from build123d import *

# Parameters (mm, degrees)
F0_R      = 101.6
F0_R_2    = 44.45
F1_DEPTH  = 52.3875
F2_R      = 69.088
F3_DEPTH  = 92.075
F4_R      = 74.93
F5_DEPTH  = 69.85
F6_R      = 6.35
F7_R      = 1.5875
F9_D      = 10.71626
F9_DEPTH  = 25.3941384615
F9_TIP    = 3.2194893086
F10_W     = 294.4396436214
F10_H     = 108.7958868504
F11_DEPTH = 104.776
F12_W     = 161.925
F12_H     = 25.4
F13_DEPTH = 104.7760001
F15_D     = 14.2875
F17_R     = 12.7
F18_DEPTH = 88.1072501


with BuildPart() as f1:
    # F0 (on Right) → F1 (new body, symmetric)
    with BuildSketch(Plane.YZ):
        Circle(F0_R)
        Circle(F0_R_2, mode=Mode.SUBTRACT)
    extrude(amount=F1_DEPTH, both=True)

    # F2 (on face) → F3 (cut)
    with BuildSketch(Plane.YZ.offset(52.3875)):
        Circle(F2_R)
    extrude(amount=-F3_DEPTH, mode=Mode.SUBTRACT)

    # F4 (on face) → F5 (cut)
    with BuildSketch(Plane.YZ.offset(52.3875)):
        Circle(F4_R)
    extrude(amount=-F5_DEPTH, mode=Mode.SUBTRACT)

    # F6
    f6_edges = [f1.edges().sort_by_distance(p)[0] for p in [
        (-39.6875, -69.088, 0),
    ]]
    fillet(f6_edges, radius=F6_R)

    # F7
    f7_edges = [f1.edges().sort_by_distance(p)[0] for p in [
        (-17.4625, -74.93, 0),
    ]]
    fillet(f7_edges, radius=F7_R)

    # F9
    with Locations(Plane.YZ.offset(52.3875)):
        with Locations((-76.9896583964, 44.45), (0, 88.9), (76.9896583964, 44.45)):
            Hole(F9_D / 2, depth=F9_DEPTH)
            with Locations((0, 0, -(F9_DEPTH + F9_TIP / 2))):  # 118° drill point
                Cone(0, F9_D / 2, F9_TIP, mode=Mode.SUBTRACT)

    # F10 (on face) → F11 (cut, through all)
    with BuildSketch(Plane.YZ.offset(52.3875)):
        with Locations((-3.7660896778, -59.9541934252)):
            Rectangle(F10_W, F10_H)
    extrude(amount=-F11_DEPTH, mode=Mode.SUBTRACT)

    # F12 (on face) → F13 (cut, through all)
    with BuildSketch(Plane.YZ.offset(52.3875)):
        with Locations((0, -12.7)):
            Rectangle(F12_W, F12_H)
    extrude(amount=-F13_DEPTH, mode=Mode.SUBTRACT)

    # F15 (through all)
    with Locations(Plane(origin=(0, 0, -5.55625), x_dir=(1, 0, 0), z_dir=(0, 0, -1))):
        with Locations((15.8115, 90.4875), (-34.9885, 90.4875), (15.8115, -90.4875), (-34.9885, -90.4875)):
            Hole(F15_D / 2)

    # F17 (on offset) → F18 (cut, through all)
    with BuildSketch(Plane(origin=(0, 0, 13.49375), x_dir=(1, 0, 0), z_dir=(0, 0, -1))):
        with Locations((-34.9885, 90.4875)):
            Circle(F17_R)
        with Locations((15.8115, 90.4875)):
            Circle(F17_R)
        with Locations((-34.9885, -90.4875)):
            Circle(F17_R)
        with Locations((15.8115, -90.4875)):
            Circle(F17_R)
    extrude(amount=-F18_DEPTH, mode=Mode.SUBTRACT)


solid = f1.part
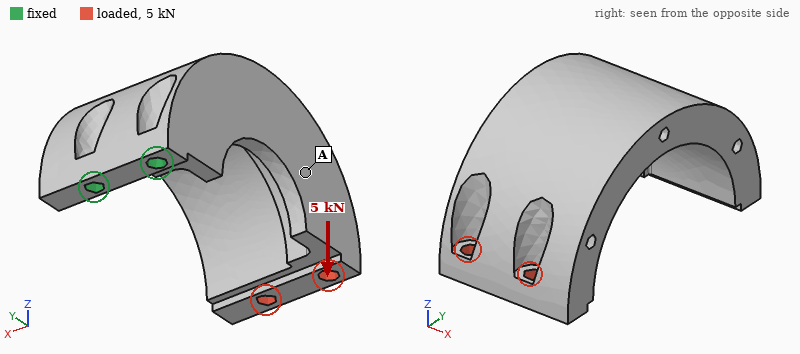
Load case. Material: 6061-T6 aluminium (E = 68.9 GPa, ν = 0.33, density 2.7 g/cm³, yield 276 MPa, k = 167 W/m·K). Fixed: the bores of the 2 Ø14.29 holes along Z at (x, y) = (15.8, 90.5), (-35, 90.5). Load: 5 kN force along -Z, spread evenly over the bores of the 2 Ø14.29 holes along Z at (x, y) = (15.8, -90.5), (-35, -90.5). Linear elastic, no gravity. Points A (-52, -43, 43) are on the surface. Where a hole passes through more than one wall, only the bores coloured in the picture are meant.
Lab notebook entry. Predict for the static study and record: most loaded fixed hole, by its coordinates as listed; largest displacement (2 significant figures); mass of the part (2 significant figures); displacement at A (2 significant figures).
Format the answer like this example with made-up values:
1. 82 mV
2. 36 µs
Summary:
1. (-35, 90.5)
2. 1.4 mm
3. 2.2 kg
4. 0.85 mm
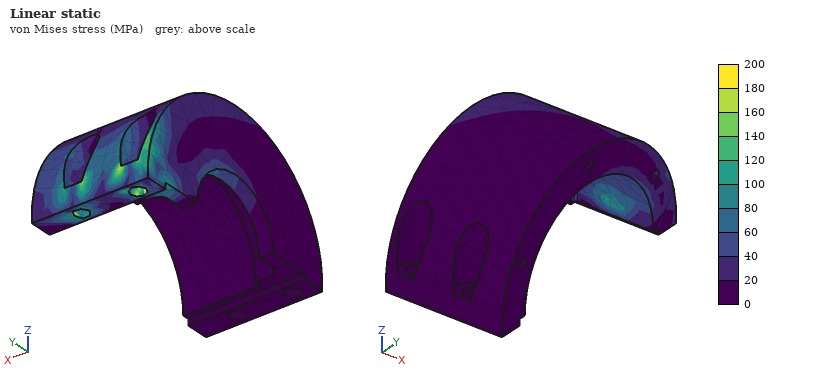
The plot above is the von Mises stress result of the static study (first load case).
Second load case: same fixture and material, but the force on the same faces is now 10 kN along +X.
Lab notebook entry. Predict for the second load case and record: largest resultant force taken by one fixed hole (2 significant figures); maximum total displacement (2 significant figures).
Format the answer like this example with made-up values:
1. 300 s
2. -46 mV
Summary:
1. 25 kN
2. 2.2 mm
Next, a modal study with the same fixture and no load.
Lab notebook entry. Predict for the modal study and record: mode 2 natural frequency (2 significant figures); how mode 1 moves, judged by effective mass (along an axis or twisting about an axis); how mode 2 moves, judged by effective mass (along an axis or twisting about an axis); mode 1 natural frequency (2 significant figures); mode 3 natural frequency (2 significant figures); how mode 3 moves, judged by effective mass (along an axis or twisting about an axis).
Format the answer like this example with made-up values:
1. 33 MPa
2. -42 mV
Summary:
1. 500 Hz
2. along Z
3. along X
4. 350 Hz
5. 1300 Hz
6. along Y
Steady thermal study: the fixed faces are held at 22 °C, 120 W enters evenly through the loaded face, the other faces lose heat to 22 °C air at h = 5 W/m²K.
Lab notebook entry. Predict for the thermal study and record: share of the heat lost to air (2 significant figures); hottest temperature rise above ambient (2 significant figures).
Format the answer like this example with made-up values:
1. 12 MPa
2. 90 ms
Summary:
1. 13 %
2. 67 K
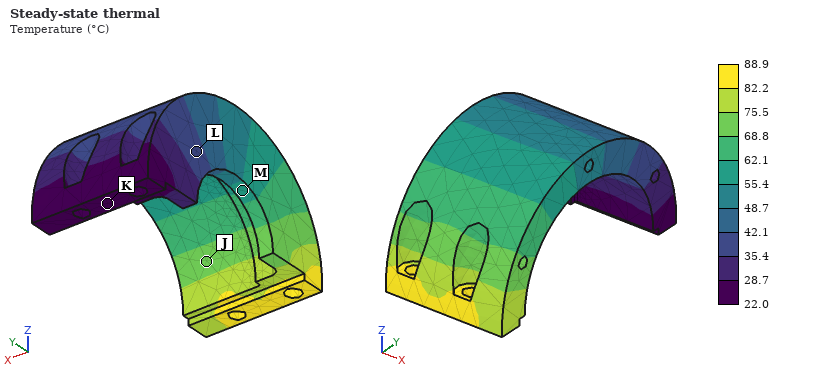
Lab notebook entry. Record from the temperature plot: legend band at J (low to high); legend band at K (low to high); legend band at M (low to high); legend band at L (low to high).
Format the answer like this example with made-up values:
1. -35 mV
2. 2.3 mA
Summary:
1. 68.8 to 75.5 °C
2. 22.0 to 28.7 °C
3. 55.4 to 62.1 °C
4. 35.4 to 42.1 °C
